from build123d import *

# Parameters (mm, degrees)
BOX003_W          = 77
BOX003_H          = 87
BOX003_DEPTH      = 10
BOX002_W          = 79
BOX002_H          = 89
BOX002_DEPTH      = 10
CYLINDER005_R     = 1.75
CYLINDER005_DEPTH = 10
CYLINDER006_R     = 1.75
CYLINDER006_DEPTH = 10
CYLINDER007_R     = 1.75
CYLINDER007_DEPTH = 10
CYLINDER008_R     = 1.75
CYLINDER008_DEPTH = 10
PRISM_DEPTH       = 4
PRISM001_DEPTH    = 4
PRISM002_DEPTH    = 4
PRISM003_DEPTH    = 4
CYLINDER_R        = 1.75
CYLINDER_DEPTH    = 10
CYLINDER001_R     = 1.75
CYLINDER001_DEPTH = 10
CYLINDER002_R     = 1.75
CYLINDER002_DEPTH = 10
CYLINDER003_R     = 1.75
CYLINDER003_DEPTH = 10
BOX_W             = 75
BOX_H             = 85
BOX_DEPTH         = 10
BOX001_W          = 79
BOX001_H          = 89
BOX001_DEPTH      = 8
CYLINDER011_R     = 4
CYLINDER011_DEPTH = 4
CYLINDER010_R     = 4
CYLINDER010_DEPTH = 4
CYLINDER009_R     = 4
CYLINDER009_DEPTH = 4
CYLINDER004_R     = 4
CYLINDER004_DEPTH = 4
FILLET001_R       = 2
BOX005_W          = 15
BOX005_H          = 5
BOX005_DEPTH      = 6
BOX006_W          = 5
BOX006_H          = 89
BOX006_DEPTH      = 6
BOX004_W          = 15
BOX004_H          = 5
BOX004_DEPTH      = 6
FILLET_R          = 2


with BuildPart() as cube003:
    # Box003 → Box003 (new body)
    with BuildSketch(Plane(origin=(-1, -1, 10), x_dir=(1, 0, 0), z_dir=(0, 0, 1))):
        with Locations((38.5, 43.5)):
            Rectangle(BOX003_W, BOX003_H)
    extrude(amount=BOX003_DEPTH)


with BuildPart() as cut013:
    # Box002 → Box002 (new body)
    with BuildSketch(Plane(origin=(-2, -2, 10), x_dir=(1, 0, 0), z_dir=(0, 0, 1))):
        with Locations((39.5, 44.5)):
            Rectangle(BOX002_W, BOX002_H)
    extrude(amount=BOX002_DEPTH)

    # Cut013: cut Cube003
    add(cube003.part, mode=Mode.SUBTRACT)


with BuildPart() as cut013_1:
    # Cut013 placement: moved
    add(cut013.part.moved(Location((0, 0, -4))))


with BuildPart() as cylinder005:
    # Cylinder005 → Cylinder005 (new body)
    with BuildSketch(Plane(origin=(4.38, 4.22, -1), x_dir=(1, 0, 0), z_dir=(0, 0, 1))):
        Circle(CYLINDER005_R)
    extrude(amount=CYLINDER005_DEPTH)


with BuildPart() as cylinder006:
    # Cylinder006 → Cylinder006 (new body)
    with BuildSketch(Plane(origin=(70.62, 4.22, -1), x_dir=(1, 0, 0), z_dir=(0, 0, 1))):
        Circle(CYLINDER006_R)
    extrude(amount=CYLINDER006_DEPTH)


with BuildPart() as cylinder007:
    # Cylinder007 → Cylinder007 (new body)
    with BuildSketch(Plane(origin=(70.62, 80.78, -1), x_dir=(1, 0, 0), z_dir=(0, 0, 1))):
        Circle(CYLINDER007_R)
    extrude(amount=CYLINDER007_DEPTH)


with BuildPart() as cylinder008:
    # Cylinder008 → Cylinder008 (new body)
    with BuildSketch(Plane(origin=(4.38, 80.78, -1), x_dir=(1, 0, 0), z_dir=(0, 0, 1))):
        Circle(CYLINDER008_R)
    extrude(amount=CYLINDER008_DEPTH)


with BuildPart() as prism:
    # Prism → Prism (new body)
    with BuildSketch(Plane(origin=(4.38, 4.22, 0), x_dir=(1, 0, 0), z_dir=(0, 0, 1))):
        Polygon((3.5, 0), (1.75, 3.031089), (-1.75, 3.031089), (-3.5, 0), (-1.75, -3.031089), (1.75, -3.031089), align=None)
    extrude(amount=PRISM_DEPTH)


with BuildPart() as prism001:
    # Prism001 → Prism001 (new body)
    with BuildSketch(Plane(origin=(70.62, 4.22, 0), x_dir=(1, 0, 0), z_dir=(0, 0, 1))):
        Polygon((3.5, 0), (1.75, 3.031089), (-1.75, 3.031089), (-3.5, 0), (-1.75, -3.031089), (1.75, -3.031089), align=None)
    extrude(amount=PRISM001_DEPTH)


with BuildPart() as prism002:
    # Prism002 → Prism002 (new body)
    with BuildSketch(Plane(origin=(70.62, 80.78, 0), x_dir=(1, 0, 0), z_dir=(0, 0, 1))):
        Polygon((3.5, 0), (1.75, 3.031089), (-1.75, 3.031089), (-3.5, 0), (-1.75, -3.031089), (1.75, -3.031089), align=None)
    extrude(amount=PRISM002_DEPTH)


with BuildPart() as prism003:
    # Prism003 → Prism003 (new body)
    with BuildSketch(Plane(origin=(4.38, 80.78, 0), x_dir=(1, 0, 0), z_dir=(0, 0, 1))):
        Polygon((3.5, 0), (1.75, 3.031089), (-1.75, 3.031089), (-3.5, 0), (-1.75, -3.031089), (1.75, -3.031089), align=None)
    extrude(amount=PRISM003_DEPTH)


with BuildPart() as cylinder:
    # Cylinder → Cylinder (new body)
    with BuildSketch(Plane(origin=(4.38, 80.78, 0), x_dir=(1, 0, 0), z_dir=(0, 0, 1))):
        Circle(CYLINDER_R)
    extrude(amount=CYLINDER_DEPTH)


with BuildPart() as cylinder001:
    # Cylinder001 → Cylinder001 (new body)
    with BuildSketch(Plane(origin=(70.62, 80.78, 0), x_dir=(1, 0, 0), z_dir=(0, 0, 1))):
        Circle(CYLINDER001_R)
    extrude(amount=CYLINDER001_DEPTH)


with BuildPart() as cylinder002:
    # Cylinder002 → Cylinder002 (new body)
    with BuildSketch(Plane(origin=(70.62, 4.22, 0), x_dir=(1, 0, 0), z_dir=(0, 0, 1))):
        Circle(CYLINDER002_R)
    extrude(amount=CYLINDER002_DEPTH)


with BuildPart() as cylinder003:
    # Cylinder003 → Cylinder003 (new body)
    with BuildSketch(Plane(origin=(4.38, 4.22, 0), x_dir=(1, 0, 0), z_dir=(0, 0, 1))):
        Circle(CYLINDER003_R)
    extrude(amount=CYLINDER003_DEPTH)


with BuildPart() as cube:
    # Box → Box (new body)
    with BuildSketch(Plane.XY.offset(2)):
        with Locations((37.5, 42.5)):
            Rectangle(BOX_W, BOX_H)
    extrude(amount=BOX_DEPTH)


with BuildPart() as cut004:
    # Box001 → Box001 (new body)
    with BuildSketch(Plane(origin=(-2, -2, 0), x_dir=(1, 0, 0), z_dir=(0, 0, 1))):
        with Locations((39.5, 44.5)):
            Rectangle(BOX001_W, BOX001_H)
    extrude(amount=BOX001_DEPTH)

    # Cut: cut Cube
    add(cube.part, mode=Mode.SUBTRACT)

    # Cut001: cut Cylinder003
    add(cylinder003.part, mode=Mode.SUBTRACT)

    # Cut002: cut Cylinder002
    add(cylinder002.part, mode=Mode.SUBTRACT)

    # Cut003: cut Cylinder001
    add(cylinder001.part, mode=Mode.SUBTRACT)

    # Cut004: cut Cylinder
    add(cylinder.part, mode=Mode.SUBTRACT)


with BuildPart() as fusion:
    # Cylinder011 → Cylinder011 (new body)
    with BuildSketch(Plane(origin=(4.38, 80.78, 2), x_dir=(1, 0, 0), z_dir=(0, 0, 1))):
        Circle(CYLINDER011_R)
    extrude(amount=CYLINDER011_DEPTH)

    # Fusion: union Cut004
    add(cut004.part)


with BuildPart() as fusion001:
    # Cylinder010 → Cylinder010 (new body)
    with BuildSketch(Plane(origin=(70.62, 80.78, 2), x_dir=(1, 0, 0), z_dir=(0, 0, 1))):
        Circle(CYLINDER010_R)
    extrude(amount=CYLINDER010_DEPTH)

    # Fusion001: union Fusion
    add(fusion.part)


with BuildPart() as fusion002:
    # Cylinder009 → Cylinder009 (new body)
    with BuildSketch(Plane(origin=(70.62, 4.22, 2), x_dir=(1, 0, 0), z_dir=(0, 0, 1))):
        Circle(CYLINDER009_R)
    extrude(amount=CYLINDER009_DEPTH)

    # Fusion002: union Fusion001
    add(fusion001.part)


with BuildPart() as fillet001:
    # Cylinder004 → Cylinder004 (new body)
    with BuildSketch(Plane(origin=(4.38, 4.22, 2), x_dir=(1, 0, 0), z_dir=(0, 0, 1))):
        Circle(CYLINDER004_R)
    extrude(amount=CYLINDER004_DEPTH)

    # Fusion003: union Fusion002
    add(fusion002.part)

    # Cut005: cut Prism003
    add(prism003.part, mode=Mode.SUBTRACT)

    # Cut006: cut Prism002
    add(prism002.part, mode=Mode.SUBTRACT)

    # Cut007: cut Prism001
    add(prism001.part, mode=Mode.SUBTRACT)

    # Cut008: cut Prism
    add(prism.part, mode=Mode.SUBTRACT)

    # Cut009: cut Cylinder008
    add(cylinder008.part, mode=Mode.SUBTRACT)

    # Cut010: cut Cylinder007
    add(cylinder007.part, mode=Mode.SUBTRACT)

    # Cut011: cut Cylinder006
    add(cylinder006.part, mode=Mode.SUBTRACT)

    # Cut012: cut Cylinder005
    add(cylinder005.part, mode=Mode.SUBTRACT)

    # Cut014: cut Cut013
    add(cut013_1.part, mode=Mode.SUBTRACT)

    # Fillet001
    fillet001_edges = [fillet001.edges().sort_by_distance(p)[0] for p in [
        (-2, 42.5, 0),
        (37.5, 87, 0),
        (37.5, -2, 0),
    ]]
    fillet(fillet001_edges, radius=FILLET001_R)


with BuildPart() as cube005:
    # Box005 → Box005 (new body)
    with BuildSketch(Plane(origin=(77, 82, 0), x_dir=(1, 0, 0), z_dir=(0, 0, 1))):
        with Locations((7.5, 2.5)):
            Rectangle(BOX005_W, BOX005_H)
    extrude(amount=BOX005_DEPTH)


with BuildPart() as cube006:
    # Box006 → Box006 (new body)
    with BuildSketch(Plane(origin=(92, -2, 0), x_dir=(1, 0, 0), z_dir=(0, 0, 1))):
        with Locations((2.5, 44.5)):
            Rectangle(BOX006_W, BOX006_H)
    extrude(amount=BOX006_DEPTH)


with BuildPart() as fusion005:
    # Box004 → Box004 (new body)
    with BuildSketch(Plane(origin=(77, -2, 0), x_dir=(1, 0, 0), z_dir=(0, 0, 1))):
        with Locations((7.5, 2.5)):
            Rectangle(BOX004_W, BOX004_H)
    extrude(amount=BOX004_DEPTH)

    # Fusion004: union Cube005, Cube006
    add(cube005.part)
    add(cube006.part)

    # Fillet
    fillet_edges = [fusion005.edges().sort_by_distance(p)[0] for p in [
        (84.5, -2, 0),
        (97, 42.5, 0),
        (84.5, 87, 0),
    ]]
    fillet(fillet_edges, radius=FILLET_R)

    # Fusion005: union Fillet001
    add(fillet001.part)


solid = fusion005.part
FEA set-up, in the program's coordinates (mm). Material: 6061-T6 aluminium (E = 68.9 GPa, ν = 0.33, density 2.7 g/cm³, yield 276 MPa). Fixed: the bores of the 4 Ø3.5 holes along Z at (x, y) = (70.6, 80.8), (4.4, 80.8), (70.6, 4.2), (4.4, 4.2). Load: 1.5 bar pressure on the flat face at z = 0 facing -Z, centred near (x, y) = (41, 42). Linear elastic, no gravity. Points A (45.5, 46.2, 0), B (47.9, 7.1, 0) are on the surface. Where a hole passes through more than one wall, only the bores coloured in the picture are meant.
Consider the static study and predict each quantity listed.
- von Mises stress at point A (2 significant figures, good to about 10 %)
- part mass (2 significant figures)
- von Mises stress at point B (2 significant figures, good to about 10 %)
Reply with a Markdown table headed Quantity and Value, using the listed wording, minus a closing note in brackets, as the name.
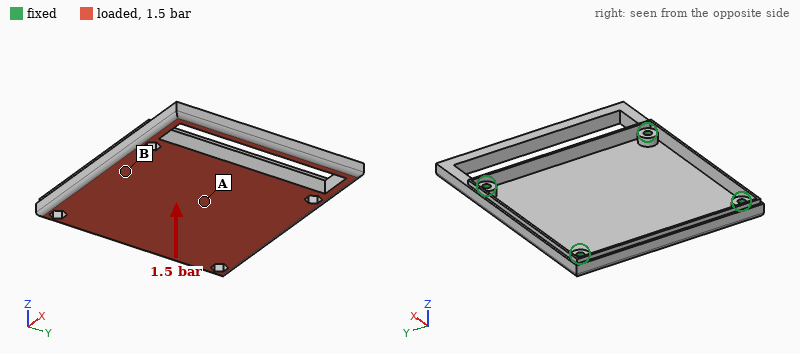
| Quantity | Value |
|---|---|
| von Mises stress at point A | 57 MPa |
| part mass | 56 g |
| von Mises stress at point B | 27 MPa |
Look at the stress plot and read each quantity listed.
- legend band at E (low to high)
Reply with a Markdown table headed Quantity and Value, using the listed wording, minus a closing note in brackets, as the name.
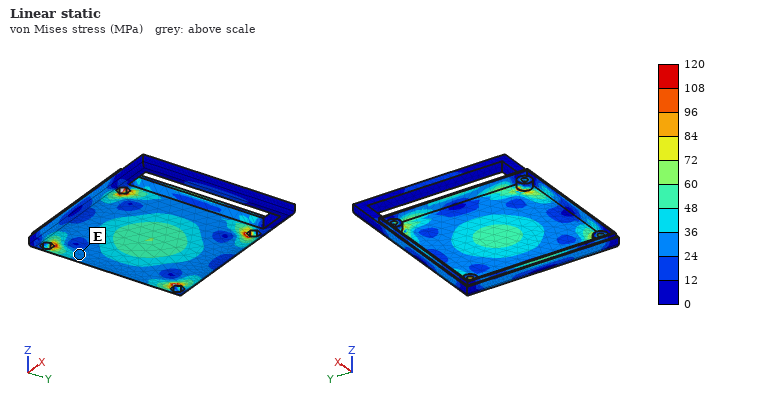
| Quantity | Value |
|---|---|
| legend band at E | 24 to 36 MPa |
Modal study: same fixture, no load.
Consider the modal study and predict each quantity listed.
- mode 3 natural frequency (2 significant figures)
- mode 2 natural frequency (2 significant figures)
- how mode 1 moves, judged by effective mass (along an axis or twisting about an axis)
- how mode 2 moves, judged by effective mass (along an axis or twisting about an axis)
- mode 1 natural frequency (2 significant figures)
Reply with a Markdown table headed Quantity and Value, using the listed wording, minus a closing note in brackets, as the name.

| Quantity | Value |
|---|---|
| mode 3 natural frequency | 3000 Hz |
| mode 2 natural frequency | 1700 Hz |
| how mode 1 moves, judged by effective mass | along Z |
| how mode 2 moves, judged by effective mass | along Z |
| mode 1 natural frequency | 1600 Hz |
